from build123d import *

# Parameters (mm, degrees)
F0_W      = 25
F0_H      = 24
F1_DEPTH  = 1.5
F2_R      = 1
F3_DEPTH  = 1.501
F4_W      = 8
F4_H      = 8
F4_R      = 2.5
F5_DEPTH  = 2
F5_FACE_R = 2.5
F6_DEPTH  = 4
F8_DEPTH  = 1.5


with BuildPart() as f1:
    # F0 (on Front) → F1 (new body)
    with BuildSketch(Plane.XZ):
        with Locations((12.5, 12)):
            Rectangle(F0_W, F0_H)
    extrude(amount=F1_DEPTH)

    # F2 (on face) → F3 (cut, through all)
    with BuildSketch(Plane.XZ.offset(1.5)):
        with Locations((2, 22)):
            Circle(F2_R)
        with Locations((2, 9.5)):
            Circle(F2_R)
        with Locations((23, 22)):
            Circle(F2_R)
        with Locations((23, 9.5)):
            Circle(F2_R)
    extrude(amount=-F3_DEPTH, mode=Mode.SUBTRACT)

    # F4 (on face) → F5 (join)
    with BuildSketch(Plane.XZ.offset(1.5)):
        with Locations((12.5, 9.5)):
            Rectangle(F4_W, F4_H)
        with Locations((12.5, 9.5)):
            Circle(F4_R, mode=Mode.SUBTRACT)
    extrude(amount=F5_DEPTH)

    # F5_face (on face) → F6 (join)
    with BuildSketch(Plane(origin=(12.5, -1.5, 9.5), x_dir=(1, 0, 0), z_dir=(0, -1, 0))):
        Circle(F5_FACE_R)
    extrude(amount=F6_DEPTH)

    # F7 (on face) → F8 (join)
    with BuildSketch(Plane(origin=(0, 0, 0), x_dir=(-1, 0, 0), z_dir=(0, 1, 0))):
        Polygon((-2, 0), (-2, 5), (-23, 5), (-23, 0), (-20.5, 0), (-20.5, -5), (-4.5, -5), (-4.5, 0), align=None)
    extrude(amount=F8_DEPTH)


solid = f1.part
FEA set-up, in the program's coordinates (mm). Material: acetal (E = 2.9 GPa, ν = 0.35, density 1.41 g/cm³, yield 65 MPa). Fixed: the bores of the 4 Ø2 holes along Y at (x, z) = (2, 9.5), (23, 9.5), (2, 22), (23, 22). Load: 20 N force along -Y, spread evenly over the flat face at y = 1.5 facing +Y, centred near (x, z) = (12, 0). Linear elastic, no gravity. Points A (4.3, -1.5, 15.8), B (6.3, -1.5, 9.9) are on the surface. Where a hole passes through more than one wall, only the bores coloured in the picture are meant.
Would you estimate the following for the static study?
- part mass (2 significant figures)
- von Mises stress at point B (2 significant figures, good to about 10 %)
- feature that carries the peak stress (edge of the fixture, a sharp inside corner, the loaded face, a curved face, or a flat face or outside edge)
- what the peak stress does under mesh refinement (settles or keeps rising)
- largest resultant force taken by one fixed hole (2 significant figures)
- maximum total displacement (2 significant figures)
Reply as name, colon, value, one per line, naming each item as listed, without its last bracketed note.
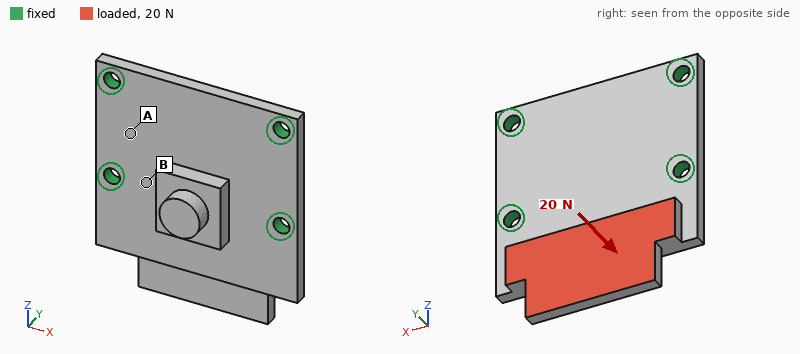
part mass: 1.9 g
von Mises stress at point B: 5.5 MPa
feature that carries the peak stress: edge of the fixture
what the peak stress does under mesh refinement: keeps rising
largest resultant force taken by one fixed hole: 14 N
maximum total displacement: 0.42 mm
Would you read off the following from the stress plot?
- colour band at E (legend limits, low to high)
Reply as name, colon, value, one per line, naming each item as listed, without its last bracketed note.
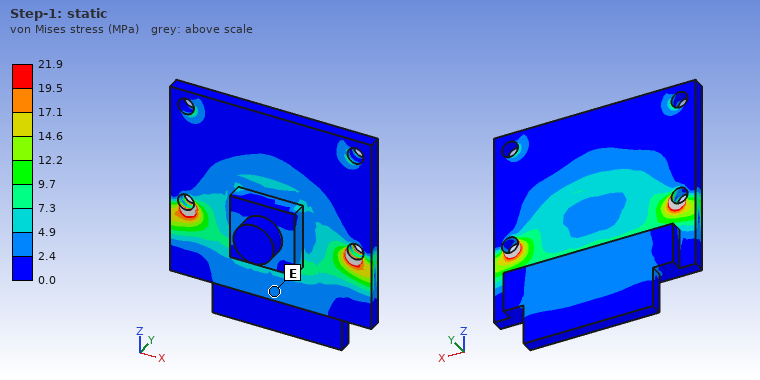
colour band at E: 2.4 to 4.9 MPa
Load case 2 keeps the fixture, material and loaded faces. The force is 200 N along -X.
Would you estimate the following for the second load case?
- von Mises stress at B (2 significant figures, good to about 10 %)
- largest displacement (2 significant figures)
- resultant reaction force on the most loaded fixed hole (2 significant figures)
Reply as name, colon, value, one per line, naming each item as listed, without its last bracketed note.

von Mises stress at B: 5.4 MPa
largest displacement: 0.18 mm
resultant reaction force on the most loaded fixed hole: 120 N
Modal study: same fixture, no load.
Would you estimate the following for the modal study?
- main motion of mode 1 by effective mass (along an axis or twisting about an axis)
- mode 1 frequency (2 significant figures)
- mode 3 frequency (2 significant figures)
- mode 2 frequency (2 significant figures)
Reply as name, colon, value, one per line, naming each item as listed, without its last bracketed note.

main motion of mode 1 by effective mass: along Y
mode 1 frequency: 1900 Hz
mode 3 frequency: 5100 Hz
mode 2 frequency: 4900 Hz
